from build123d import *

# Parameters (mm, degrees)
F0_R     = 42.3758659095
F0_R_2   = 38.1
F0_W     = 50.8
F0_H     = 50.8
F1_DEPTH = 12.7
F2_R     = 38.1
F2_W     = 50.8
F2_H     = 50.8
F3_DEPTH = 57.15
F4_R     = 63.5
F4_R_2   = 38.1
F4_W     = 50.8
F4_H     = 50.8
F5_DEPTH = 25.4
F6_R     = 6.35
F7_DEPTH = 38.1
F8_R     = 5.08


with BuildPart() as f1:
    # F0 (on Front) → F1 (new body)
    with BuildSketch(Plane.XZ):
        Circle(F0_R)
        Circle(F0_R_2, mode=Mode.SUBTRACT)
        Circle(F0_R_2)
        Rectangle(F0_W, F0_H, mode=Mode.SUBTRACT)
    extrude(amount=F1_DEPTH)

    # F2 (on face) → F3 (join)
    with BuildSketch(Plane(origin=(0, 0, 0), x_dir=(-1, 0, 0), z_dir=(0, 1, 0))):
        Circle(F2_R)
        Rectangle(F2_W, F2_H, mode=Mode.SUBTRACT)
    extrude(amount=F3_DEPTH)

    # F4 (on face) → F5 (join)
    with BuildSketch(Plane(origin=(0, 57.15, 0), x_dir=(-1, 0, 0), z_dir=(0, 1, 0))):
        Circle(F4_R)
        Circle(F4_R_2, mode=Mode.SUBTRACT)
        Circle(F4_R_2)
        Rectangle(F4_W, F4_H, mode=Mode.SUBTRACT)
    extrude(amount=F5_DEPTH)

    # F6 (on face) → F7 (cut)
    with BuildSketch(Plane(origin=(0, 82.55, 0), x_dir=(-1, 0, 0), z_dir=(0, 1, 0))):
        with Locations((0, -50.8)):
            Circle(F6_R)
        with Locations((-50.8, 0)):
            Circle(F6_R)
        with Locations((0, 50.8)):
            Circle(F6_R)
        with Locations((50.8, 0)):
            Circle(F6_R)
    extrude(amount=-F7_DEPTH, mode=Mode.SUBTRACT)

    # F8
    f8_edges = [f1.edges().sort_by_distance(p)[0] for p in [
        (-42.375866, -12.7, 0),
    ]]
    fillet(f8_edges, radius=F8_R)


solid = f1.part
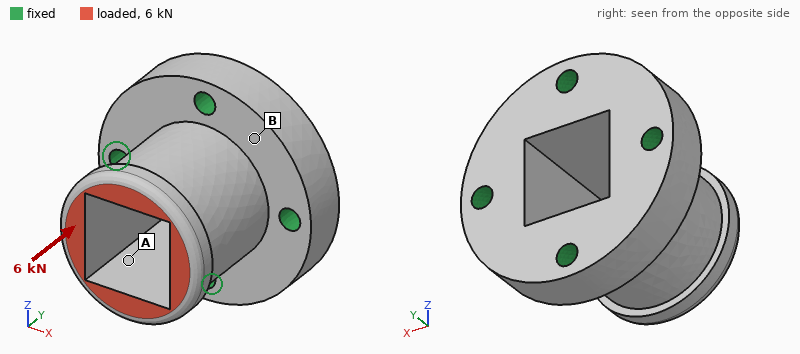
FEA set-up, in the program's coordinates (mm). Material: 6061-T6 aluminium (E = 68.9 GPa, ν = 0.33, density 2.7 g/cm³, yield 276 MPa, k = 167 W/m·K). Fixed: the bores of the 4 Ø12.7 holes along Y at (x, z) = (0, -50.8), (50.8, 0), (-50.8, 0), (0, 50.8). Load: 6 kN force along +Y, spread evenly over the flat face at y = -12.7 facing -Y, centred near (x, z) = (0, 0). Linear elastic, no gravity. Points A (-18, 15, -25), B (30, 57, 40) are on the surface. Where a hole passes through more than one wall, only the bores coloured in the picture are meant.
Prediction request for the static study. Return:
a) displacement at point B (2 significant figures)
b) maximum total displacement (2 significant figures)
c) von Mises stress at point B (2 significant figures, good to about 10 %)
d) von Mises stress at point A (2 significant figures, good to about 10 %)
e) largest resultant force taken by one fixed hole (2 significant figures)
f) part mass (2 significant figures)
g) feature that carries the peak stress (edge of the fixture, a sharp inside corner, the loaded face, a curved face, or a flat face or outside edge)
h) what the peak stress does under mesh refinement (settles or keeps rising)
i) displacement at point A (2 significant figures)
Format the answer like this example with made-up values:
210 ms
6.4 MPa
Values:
0.82 µm
4.8 µm
1.1 MPa
3.2 MPa
1.5 kN
1.1 kg
edge of the fixture
keeps rising
3.3 µm
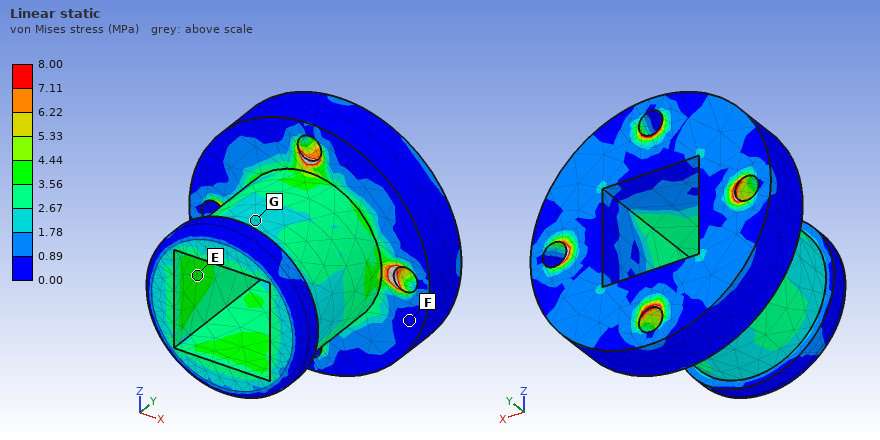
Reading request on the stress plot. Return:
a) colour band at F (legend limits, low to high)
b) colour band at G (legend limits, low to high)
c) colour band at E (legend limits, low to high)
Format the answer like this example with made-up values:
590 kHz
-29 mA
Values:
0.00 to 0.89 MPa
1.78 to 2.67 MPa
3.56 to 4.44 MPa
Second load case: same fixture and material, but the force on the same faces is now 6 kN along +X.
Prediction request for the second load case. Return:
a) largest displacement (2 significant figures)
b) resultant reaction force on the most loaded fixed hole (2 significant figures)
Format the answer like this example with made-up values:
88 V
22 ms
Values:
53 µm
5.2 kN
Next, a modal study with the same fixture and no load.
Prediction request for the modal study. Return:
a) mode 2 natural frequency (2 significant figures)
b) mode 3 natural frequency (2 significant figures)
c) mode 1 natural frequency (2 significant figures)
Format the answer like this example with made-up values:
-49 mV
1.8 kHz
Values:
4700 Hz
4900 Hz
4700 Hz
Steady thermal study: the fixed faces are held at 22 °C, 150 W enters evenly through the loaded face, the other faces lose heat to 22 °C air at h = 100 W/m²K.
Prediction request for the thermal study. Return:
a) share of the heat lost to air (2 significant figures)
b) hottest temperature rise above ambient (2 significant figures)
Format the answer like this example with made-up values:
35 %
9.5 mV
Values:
36 %
28 K
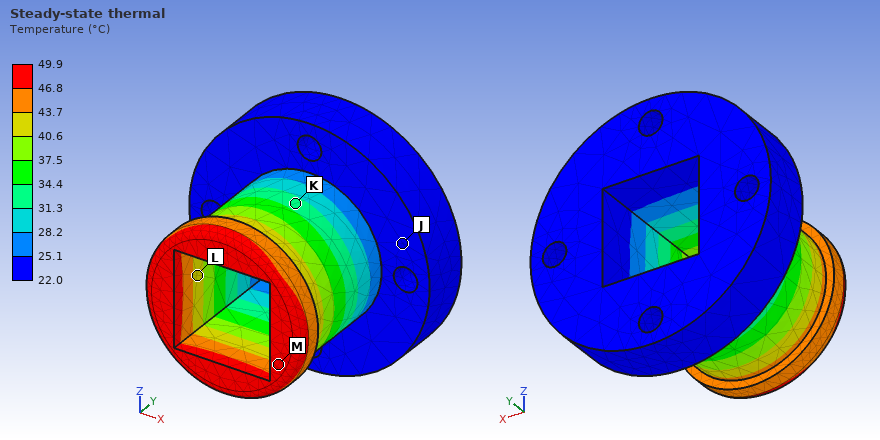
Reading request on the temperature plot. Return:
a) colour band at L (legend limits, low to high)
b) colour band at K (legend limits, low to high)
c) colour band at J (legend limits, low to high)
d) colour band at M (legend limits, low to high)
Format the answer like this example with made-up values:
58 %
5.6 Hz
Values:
40.6 to 43.7 °C
31.3 to 34.4 °C
22.0 to 25.1 °C
46.8 to 49.9 °C
